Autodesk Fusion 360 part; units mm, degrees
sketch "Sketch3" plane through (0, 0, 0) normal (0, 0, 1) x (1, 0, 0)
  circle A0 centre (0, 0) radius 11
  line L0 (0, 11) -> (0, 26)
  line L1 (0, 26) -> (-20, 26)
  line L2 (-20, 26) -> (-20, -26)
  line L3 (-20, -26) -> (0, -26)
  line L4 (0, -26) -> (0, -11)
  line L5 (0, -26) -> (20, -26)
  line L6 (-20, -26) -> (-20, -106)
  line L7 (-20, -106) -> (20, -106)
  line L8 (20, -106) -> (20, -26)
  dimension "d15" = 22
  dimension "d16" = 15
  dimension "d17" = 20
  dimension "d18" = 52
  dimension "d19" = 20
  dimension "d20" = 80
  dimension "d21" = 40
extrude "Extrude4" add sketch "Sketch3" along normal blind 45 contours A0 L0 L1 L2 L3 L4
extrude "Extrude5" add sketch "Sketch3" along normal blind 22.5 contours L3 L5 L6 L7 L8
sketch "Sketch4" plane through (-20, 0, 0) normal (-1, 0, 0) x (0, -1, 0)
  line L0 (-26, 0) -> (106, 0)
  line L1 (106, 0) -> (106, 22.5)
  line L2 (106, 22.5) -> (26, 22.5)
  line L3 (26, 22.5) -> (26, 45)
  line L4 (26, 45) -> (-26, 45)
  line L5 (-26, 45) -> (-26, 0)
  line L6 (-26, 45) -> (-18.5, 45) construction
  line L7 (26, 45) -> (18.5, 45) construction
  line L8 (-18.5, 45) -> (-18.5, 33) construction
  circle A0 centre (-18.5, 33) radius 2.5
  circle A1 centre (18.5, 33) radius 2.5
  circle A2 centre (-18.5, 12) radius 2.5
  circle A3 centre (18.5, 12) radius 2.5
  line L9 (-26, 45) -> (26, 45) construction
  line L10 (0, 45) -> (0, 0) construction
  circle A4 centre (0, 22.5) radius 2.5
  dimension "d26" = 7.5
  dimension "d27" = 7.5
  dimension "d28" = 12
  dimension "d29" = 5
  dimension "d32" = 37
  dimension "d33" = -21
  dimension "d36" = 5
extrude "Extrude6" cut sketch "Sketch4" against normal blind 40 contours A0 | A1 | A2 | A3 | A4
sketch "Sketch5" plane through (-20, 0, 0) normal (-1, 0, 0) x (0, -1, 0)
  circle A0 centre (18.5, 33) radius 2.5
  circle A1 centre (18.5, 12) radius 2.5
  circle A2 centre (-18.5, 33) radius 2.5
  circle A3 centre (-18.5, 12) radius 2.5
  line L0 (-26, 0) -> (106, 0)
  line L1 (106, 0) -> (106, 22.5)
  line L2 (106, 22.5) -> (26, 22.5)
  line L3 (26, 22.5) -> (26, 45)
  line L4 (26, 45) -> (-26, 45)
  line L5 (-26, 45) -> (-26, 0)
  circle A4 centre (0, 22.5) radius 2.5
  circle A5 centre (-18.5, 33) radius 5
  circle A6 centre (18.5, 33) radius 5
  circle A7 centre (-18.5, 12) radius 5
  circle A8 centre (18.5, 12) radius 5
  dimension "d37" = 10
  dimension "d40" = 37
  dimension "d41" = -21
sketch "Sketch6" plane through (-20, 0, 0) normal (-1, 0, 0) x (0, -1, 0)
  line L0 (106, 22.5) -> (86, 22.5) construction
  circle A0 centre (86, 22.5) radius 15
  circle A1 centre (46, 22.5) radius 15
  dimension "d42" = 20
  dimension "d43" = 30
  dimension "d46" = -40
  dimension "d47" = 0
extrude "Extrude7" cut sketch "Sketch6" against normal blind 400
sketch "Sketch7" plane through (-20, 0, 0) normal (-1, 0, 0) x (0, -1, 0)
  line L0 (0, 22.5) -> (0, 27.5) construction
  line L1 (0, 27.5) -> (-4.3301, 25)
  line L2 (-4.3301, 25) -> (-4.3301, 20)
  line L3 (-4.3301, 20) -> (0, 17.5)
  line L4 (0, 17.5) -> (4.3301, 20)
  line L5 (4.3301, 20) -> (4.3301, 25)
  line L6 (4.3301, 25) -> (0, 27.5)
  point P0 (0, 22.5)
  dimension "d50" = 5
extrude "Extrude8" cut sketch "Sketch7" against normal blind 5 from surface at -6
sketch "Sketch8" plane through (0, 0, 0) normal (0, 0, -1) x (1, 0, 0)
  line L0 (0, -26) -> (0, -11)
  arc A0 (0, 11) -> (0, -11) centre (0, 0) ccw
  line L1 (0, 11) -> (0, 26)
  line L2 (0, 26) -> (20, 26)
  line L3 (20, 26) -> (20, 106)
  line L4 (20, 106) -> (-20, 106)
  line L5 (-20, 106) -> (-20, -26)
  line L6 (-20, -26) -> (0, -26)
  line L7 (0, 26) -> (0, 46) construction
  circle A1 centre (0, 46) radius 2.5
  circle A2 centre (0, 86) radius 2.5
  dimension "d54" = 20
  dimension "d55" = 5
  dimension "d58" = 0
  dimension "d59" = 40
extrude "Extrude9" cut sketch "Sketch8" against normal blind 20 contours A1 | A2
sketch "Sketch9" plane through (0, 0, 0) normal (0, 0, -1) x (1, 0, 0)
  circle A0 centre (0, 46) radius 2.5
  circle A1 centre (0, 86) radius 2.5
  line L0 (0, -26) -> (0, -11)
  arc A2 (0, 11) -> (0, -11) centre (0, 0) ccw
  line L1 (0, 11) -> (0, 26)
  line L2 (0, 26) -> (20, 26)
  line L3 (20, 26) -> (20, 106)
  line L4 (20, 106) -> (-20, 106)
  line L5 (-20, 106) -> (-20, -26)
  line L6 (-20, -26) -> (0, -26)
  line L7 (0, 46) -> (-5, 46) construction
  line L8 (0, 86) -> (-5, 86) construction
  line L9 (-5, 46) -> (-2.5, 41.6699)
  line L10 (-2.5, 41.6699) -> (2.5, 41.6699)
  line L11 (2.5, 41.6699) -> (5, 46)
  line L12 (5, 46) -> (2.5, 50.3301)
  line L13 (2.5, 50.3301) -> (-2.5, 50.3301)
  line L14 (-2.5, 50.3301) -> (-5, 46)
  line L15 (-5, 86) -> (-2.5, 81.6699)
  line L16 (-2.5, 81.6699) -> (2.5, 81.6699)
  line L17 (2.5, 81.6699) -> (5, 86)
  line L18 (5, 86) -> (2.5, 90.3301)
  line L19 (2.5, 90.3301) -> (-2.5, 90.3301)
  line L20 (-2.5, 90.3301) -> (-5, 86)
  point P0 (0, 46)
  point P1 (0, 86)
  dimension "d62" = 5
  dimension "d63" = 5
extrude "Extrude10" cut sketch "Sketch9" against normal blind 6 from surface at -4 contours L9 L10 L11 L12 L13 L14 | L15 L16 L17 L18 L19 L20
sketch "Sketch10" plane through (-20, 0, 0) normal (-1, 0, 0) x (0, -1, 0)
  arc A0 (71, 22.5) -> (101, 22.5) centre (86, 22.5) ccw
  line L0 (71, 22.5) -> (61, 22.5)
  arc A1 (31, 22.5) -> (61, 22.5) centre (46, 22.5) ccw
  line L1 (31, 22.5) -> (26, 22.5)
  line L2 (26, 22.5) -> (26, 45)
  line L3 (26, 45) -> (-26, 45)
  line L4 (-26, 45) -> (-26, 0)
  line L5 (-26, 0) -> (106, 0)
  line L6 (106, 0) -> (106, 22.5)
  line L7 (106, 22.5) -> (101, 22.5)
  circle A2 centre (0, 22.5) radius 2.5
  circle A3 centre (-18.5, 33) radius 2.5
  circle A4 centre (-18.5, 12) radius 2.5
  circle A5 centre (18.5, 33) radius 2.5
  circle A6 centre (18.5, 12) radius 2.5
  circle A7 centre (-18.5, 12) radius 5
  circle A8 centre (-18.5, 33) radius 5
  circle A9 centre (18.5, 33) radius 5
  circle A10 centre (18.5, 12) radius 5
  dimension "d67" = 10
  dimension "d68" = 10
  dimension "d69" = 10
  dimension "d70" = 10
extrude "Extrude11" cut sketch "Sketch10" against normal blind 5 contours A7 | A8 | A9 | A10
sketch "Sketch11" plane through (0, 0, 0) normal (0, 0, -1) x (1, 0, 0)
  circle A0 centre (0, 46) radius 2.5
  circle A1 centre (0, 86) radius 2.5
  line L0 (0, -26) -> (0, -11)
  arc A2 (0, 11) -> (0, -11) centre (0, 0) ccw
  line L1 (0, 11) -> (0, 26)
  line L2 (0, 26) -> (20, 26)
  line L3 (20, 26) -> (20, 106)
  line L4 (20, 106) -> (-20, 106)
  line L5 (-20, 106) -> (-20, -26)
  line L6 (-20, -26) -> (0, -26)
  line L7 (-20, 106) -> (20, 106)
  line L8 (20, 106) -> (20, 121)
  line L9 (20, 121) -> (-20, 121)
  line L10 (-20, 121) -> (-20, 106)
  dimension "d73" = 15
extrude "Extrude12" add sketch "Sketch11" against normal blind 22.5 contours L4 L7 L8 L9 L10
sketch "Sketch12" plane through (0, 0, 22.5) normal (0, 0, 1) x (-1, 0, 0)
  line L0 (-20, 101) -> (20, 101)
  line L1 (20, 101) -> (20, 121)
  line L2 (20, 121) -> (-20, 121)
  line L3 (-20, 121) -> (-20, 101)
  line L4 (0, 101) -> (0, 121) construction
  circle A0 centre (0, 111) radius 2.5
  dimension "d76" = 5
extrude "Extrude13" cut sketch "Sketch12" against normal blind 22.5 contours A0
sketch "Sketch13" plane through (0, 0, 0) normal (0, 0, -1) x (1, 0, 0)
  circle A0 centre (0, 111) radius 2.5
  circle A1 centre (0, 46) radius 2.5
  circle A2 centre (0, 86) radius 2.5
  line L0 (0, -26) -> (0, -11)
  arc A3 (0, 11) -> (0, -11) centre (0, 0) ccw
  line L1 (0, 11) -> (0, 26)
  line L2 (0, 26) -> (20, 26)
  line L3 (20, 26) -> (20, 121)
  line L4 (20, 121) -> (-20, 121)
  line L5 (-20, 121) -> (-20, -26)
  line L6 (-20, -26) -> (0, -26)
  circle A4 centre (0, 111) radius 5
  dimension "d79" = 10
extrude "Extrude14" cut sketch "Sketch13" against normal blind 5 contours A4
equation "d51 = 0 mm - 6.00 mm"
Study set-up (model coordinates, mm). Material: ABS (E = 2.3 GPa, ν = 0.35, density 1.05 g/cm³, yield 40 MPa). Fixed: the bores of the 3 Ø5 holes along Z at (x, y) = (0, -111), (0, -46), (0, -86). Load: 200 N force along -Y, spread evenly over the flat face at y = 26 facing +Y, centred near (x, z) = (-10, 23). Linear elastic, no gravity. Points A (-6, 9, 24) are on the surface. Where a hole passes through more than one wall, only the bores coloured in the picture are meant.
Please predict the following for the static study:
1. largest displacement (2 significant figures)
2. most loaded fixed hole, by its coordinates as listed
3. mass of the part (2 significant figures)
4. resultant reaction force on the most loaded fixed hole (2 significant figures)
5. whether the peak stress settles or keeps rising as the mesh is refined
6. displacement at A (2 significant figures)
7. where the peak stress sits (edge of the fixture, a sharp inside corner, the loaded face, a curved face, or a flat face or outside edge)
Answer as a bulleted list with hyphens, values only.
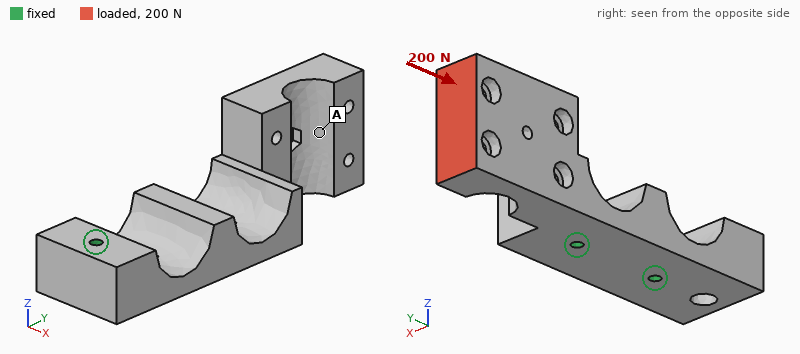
- 1.5 mm
- (0, -86)
- 96 g
- 180 N
- keeps rising
- 1.0 mm
- edge of the fixture
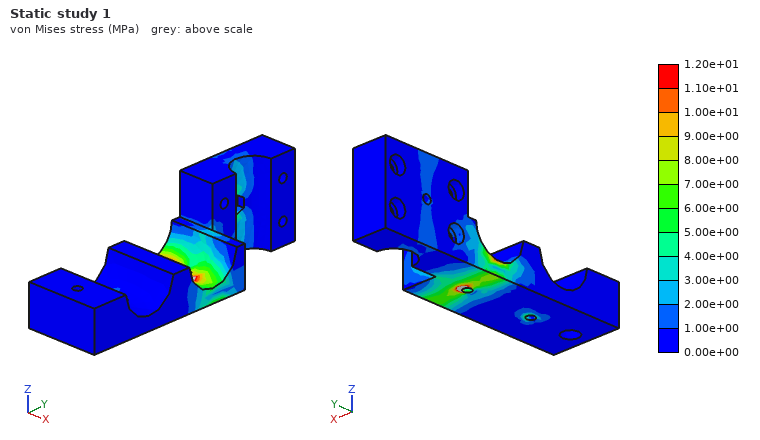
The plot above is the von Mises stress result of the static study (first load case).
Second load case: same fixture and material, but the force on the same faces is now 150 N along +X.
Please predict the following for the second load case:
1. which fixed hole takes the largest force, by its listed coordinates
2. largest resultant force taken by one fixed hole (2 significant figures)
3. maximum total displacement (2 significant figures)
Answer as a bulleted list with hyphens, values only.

- (0, -46)
- 350 N
- 1.6 mm
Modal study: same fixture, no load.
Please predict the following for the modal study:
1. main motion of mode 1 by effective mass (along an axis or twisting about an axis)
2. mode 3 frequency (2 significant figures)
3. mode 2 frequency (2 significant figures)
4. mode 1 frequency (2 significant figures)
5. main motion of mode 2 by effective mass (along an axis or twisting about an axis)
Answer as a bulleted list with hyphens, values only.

- along Z
- 850 Hz
- 410 Hz
- 230 Hz
- along X
